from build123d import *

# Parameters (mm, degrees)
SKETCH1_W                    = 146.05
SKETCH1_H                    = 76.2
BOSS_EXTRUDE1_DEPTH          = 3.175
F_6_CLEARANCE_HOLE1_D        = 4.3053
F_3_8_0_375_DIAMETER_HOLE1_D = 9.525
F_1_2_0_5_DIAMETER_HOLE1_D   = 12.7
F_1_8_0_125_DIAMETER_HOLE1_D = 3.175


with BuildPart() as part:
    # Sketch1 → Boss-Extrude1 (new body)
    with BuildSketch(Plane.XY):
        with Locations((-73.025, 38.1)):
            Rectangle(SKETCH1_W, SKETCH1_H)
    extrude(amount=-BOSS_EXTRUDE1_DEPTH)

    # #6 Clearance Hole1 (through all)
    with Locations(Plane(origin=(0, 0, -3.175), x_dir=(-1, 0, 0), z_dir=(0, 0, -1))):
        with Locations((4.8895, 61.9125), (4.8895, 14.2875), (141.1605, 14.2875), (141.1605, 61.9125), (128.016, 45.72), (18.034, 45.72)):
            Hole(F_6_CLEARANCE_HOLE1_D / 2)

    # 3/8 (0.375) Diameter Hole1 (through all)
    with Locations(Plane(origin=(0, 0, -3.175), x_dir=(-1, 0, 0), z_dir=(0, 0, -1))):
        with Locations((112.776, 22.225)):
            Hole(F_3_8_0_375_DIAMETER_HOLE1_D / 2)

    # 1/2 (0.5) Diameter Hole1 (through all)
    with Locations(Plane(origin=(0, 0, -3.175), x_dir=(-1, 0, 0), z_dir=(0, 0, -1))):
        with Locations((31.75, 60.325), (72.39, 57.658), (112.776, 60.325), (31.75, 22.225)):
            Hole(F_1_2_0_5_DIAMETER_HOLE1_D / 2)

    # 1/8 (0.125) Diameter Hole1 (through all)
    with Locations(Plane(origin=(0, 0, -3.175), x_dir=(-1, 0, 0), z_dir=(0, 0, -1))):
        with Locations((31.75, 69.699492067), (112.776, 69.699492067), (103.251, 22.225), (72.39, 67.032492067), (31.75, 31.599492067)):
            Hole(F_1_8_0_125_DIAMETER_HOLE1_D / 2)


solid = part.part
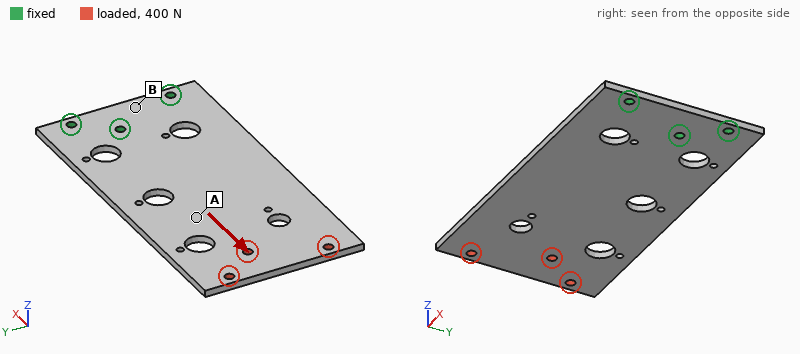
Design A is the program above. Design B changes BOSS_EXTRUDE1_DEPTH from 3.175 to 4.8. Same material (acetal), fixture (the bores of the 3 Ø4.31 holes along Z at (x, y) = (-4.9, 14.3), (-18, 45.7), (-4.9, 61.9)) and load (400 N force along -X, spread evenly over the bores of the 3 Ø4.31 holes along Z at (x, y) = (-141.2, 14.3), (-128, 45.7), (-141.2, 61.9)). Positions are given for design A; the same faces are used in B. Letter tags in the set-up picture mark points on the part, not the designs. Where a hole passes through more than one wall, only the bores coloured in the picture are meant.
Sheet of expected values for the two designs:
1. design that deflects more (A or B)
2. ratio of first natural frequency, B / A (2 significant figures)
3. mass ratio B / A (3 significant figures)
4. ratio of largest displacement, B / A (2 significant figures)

A
1.5
1.51
0.66
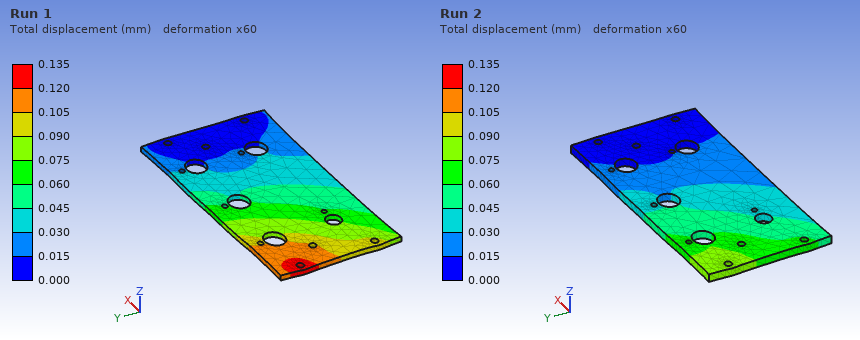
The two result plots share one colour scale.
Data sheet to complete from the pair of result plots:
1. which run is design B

Run 2
